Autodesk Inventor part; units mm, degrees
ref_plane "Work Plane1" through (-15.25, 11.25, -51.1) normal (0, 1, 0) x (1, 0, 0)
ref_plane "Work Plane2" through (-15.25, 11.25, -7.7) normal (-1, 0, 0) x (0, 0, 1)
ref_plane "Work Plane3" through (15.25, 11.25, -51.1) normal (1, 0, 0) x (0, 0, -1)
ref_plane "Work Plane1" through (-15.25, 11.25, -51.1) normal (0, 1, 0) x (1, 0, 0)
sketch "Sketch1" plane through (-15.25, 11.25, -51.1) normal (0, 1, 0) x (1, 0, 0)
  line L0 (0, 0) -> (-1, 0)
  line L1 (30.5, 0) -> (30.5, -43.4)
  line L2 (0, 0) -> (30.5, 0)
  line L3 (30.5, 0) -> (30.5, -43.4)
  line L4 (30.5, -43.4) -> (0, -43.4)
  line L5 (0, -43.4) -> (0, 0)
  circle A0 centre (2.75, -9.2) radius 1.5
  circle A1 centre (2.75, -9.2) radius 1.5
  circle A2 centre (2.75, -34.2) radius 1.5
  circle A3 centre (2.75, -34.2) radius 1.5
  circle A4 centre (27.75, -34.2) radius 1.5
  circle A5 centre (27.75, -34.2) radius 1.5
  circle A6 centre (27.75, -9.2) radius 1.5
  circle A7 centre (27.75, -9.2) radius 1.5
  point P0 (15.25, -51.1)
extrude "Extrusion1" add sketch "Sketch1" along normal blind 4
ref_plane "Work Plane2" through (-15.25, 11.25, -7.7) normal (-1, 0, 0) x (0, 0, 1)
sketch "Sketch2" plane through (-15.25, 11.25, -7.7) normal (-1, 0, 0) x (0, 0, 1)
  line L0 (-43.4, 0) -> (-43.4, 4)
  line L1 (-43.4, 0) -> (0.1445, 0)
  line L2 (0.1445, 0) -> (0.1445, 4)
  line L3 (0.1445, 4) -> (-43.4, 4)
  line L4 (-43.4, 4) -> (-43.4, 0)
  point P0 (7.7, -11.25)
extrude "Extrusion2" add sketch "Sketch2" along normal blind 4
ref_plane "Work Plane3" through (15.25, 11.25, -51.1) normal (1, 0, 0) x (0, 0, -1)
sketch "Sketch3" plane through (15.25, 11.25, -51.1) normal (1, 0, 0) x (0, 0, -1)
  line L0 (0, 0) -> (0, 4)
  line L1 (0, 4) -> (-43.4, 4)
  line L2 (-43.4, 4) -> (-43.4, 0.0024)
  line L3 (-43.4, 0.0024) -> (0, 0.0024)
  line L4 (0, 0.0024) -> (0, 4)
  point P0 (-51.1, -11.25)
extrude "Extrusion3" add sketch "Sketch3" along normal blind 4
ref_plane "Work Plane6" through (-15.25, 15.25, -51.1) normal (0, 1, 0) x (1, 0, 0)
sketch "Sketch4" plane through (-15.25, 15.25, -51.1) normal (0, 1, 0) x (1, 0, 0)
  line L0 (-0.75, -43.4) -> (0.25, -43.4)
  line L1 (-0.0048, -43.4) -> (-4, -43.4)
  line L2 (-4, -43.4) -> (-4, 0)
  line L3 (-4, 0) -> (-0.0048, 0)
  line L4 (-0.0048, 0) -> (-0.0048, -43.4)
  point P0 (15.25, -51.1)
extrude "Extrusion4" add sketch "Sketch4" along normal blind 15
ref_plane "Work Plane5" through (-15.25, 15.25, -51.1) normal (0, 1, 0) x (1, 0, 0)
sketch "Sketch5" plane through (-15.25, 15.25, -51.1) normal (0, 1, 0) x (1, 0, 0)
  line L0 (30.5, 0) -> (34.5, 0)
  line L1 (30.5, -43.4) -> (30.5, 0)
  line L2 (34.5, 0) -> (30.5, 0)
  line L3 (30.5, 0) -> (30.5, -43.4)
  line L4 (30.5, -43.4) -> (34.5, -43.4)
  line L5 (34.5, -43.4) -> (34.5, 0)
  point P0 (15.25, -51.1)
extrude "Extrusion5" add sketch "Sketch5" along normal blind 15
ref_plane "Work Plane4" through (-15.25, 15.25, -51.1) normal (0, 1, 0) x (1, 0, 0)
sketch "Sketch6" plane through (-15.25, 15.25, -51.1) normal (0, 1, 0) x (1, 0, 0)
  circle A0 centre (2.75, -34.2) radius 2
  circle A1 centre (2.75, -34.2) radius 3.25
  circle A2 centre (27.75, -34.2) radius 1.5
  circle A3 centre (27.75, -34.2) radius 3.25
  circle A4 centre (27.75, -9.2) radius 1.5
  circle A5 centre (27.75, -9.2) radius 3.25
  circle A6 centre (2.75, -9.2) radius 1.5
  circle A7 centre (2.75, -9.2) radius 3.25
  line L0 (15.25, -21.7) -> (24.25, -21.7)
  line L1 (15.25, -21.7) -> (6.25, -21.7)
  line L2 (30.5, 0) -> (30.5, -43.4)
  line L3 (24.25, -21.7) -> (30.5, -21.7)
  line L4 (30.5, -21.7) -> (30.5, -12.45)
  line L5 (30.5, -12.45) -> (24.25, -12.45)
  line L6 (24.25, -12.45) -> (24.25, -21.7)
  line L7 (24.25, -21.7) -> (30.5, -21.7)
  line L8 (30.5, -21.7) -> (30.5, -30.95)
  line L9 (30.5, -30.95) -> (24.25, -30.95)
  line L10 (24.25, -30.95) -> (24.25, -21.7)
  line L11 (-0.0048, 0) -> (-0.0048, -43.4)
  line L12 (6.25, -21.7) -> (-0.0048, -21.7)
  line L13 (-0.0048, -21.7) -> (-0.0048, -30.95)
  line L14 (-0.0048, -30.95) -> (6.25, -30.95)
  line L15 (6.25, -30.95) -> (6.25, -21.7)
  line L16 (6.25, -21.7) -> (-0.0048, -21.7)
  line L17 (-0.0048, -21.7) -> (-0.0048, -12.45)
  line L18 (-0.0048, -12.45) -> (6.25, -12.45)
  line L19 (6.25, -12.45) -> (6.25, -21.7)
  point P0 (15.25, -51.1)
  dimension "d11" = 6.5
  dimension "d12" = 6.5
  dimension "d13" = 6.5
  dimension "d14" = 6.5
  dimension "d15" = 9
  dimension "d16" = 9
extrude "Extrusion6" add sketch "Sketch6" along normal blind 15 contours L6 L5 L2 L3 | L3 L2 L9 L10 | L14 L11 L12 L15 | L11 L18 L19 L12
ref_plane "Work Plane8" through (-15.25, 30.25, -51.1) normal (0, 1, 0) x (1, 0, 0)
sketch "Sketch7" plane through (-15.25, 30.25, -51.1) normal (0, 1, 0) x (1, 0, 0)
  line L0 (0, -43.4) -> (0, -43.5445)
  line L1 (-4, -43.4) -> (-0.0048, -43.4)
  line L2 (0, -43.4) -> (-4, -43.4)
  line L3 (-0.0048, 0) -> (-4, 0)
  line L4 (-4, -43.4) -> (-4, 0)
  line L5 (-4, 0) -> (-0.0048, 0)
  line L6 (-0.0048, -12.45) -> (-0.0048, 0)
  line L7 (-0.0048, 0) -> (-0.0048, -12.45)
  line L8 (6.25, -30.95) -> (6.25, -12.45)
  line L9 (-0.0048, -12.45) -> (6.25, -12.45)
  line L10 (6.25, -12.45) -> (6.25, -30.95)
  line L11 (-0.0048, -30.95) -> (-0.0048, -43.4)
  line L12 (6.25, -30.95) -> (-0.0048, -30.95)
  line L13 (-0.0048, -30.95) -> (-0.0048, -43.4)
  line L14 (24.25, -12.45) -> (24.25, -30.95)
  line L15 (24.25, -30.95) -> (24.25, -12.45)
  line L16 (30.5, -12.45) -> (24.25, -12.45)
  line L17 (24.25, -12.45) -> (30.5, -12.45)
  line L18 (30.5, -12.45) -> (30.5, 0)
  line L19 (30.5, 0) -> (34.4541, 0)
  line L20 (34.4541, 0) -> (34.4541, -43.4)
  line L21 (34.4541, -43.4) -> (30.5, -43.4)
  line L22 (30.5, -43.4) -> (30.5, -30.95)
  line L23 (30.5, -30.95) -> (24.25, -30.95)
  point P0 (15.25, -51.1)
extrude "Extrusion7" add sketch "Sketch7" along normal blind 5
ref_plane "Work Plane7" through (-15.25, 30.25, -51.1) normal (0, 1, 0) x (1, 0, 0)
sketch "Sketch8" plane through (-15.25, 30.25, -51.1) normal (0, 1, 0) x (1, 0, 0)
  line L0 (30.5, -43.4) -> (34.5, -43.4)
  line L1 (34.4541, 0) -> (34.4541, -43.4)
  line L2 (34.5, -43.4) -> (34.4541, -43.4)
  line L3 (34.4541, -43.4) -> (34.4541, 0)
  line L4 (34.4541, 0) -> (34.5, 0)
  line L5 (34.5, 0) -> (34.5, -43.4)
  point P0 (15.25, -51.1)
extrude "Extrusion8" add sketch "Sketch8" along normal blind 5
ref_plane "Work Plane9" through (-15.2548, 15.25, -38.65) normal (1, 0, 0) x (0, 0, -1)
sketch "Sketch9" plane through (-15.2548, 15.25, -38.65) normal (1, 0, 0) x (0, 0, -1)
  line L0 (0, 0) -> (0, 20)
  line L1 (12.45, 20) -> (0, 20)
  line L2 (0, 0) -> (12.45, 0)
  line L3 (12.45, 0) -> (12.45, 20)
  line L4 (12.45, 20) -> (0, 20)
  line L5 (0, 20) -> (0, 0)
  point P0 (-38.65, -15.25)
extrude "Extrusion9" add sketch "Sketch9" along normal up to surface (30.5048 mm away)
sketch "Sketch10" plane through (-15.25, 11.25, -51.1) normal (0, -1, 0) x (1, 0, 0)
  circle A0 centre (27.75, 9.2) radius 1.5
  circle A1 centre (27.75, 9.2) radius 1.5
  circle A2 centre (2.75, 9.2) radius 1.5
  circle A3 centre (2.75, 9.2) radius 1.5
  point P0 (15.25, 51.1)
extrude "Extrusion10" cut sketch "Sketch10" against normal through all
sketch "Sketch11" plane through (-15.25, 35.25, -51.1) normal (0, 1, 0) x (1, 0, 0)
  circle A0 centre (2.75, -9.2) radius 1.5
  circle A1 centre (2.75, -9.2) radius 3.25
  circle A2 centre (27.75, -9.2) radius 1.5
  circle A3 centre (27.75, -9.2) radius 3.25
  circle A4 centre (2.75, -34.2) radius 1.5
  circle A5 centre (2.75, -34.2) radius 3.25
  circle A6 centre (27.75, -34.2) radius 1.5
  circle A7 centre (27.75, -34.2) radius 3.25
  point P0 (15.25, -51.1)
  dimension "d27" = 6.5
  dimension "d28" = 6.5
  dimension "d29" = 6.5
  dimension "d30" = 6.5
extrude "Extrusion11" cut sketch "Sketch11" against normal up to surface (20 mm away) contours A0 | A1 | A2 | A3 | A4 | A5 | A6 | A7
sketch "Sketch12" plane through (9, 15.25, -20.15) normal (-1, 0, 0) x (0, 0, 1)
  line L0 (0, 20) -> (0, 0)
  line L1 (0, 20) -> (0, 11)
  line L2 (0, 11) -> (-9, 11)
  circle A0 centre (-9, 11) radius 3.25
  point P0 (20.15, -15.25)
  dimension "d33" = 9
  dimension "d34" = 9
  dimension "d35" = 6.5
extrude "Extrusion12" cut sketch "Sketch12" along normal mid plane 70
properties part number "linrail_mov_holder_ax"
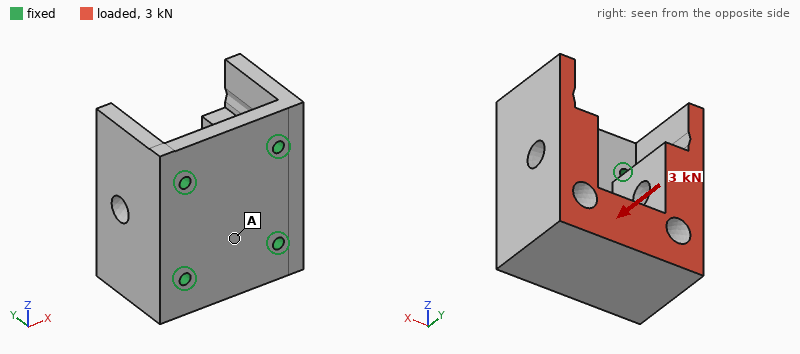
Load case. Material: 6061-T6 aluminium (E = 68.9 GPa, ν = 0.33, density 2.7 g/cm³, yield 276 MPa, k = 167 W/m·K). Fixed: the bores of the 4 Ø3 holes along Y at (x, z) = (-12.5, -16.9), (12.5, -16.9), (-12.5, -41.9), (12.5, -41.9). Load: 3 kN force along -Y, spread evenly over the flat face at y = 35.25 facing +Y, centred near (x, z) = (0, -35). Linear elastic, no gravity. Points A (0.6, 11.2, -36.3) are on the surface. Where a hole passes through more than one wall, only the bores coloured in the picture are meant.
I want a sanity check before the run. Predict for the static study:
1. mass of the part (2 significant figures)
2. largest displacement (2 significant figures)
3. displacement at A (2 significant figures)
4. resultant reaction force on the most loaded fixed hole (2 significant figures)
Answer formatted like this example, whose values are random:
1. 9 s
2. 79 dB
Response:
1. 64 g
2. 4.6 µm
3. 2.8 µm
4. 1.1 kN
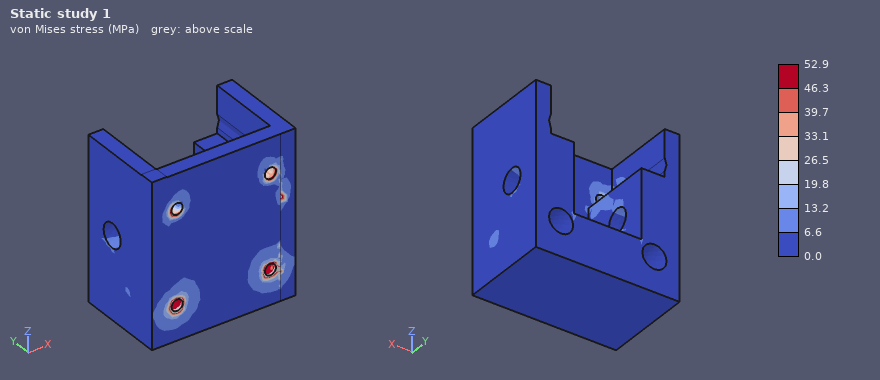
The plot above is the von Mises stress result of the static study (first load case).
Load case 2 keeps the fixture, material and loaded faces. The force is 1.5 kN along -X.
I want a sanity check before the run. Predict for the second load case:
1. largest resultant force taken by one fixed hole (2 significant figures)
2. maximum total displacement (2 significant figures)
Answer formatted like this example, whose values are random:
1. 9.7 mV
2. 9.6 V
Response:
1. 1.2 kN
2. 33 µm
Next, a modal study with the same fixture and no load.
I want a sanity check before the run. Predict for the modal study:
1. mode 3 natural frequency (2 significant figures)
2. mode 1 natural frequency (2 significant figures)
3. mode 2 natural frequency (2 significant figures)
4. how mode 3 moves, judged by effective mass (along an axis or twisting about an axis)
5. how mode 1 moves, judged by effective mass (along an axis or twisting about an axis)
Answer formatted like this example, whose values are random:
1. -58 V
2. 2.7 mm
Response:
1. 14 kHz
2. 10 kHz
3. 11 kHz
4. along Z
5. along X
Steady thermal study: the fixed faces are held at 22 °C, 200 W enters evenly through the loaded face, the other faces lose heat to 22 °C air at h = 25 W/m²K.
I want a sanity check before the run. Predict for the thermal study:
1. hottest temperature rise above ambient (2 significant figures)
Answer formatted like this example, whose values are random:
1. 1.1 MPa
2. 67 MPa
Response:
1. 49 K
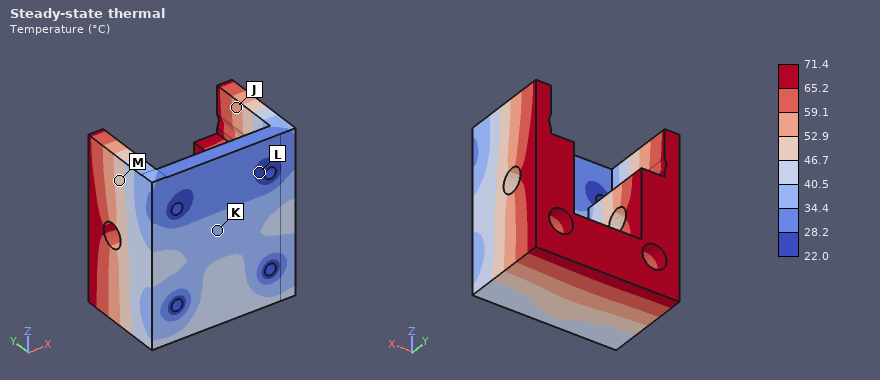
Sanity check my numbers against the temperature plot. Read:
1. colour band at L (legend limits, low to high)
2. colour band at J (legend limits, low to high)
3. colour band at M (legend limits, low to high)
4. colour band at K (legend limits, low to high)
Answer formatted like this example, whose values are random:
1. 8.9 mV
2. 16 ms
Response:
1. 22.0 to 28.2 °C
2. 52.9 to 59.1 °C
3. 46.7 to 52.9 °C
4. 34.4 to 40.5 °C
